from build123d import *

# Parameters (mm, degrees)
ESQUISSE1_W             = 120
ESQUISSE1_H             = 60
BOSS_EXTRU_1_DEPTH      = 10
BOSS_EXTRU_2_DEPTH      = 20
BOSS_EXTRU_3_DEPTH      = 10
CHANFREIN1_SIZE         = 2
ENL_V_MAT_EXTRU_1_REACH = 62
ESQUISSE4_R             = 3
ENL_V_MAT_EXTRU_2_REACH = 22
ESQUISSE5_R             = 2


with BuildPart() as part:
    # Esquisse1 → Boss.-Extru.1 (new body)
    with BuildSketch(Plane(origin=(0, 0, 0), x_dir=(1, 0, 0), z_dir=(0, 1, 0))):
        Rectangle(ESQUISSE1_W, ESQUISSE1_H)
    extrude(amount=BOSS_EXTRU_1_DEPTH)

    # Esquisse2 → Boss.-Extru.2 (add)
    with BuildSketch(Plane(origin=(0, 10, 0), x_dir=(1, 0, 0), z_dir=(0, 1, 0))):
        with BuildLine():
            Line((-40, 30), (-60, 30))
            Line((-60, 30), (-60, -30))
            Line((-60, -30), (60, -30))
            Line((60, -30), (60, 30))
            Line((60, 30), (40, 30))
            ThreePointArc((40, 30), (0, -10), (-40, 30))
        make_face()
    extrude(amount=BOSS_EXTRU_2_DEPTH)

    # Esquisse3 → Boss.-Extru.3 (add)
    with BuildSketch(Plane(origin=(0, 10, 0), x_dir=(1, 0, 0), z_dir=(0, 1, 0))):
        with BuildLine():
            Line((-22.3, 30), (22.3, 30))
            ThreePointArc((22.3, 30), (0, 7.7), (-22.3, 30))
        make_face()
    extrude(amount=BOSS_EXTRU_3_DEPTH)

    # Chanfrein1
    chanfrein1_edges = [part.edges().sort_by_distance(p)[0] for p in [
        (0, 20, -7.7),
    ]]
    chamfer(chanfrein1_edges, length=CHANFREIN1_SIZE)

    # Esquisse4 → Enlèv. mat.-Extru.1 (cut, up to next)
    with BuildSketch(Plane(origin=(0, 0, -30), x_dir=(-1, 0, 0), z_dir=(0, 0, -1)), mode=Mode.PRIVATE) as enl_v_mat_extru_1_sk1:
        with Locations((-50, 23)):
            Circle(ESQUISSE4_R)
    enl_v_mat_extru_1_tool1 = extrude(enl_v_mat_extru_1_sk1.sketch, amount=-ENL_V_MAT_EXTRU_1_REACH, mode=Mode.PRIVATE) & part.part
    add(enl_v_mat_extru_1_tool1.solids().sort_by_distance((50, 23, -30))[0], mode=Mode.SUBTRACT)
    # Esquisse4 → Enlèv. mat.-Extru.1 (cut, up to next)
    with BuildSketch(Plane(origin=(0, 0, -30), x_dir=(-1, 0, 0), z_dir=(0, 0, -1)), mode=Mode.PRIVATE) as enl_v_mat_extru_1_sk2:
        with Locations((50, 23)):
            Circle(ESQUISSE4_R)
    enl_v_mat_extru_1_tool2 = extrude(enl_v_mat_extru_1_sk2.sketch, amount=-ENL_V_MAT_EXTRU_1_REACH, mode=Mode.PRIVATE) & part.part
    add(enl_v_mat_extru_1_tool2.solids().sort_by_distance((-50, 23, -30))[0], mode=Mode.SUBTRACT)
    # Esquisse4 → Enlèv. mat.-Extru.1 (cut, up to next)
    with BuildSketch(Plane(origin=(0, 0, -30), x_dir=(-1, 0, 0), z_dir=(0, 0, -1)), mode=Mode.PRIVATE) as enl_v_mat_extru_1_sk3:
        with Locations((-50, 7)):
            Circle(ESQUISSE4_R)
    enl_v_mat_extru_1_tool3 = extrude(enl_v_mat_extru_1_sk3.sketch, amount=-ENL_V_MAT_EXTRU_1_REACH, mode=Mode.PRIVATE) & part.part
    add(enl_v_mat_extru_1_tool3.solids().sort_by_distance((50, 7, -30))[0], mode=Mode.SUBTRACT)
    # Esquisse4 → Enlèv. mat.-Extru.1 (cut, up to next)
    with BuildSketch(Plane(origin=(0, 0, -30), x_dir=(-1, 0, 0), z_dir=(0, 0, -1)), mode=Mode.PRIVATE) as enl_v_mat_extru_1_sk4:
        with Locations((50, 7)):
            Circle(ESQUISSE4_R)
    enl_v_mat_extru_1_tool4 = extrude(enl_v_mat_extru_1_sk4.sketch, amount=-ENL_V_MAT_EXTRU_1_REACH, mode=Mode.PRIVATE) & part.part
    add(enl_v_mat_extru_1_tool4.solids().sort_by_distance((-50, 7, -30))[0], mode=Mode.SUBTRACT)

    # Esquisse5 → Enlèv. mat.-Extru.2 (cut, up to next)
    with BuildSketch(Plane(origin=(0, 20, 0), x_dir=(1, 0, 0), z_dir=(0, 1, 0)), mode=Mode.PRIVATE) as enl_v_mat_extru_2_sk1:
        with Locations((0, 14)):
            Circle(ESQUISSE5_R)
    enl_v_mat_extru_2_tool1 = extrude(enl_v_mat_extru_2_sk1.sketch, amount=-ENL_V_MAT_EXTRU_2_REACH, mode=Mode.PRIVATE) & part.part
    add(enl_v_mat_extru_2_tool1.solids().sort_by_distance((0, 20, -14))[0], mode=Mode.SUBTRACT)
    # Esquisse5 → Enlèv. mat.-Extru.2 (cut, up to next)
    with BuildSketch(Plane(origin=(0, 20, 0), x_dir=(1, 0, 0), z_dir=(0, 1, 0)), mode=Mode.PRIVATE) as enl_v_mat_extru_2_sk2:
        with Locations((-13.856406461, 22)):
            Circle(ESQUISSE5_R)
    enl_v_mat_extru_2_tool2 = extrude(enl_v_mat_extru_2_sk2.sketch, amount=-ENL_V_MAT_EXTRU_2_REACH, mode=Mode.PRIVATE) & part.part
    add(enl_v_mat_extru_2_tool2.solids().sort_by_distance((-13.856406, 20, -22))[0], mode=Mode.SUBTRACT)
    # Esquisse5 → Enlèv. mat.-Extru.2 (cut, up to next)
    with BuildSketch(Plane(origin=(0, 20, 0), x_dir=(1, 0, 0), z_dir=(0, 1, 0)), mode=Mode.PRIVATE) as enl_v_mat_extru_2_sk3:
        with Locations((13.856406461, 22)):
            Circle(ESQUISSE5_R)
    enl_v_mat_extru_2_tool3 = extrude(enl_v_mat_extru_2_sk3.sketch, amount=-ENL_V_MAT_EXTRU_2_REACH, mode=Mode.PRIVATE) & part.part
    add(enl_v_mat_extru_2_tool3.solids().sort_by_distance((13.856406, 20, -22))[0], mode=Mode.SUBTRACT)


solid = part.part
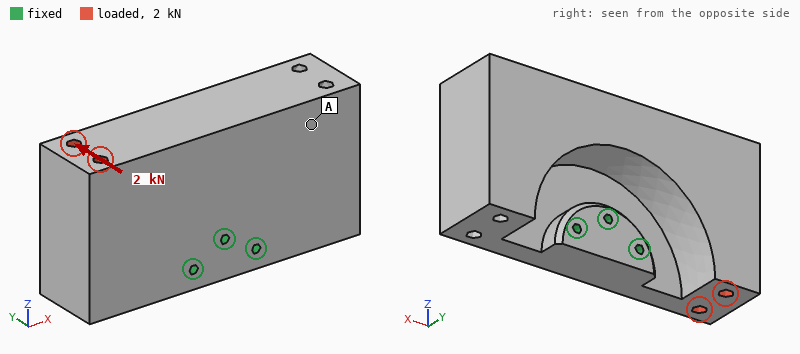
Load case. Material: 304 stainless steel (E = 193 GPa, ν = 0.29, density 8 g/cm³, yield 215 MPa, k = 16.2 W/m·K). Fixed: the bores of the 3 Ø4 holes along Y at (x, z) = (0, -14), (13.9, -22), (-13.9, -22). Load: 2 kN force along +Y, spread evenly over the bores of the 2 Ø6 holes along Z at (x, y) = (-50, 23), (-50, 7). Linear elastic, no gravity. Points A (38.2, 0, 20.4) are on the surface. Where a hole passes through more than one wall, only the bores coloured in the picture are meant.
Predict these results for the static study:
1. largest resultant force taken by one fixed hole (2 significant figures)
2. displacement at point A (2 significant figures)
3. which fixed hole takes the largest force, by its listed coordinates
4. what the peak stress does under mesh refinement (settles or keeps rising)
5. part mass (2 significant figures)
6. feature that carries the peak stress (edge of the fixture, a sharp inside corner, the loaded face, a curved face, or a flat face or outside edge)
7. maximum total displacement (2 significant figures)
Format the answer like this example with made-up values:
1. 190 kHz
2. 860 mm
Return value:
1. 2.2 kN
2. 8.0 µm
3. (-13.9, -22)
4. keeps rising
5. 1.3 kg
6. edge of the fixture
7. 49 µm
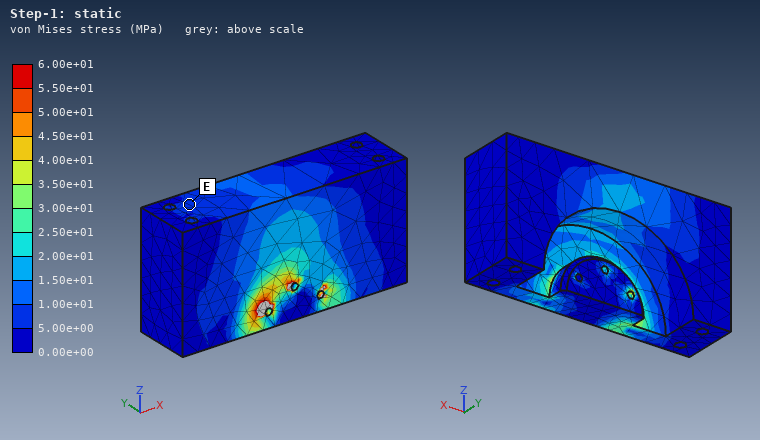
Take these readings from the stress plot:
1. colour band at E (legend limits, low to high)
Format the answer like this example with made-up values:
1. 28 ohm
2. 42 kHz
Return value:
1. 5.00e+00 to 1.00e+01 MPa
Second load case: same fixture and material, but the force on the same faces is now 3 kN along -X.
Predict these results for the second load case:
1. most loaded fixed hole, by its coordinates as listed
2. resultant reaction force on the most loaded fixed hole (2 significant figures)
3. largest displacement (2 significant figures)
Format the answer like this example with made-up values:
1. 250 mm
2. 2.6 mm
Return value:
1. (0, -14)
2. 2.1 kN
3. 15 µm
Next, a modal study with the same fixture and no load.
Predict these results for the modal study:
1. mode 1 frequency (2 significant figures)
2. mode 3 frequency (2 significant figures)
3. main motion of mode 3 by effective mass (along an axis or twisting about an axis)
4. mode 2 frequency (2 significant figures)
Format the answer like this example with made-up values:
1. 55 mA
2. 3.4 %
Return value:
1. 1700 Hz
2. 2800 Hz
3. along X
4. 1700 Hz
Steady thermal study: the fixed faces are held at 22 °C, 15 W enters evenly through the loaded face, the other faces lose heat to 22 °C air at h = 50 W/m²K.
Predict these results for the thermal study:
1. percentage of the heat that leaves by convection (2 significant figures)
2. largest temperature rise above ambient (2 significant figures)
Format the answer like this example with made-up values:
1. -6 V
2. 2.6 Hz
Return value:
1. 73 %
2. 23 K
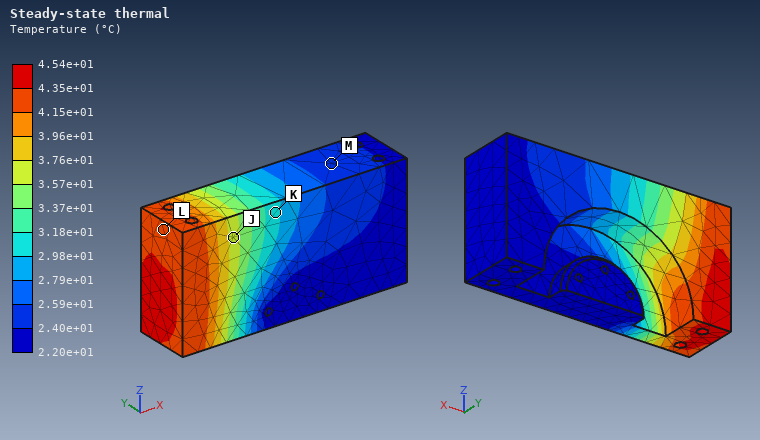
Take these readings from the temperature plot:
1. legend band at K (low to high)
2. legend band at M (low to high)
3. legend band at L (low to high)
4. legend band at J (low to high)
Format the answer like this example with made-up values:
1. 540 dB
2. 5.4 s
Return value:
1. 2.98e+01 to 3.18e+01 °C
2. 2.40e+01 to 2.59e+01 °C
3. 4.15e+01 to 4.35e+01 °C
4. 3.57e+01 to 3.76e+01 °C
